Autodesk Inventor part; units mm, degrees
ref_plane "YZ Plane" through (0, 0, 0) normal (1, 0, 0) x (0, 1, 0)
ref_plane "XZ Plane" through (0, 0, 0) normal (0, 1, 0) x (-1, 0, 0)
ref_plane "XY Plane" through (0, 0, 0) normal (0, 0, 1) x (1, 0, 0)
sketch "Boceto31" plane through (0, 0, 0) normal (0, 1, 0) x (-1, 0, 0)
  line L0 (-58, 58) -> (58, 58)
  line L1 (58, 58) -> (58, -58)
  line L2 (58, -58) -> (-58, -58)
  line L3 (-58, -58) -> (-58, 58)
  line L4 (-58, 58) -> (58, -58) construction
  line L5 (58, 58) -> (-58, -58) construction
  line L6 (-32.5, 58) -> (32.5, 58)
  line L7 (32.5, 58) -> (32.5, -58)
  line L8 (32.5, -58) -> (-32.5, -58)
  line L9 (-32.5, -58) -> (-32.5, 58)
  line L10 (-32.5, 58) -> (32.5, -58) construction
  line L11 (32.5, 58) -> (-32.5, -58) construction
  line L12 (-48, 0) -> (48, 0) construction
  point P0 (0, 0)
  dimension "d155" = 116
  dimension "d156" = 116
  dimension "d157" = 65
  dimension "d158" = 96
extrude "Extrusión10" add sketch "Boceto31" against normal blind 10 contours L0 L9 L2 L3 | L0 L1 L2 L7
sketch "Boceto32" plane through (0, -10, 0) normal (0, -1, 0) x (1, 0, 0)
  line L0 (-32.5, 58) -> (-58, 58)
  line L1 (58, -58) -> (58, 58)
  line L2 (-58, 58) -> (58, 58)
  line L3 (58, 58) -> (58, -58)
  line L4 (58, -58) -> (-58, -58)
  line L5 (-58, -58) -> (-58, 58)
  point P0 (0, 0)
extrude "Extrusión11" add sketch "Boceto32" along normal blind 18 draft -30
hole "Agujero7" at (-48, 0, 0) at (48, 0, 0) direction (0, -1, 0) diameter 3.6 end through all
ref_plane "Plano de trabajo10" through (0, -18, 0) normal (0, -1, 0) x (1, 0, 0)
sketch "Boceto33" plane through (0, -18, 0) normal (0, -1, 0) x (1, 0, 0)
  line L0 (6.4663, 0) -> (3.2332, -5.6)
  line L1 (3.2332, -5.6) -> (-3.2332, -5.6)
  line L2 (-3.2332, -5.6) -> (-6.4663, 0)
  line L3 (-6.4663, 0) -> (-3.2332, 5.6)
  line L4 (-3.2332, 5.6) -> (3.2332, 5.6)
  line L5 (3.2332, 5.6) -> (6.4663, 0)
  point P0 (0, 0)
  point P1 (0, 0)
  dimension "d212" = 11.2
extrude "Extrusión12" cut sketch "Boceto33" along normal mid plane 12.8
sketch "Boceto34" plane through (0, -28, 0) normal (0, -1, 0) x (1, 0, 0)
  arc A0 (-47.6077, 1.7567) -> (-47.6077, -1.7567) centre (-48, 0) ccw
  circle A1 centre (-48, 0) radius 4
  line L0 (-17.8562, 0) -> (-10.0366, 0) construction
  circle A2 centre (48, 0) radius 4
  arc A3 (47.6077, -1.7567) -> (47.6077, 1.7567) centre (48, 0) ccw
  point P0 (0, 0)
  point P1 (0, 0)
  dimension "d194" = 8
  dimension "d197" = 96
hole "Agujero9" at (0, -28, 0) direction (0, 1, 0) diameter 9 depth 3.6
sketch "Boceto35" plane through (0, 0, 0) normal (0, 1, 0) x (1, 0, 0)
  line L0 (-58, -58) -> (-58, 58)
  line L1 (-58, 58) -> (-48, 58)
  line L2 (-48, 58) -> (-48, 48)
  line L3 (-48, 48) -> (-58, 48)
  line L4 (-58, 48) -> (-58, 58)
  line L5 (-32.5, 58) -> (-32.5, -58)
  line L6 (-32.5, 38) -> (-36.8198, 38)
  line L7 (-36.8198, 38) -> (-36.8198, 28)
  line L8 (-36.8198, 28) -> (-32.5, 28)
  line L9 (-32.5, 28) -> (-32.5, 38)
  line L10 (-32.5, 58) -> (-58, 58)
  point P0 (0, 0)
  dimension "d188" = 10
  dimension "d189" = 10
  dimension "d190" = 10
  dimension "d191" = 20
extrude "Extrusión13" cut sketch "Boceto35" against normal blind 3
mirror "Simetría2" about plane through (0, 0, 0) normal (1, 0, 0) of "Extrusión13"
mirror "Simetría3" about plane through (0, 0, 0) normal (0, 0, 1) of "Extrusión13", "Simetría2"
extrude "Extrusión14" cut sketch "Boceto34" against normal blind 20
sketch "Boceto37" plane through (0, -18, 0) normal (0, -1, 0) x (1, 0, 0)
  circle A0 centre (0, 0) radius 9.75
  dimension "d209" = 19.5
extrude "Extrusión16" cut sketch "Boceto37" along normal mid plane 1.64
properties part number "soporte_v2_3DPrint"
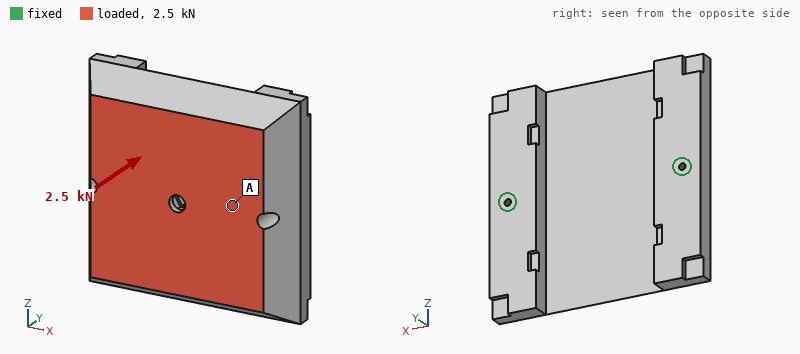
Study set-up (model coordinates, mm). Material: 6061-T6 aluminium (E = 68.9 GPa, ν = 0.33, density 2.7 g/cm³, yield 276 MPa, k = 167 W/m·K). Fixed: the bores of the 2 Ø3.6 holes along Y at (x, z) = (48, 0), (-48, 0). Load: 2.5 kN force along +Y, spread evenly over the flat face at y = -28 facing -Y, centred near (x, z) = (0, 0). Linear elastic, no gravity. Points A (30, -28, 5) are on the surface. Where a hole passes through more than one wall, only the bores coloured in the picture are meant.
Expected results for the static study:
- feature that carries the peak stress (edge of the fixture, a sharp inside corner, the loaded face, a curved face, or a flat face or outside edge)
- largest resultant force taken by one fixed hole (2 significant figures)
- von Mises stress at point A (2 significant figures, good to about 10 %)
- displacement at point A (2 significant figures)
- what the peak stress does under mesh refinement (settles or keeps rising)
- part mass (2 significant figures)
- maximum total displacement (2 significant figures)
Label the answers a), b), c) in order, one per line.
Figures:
a) edge of the fixture
b) 1.6 kN
c) 3.1 MPa
d) 4.3 µm
e) keeps rising
f) 690 g
g) 9.5 µm
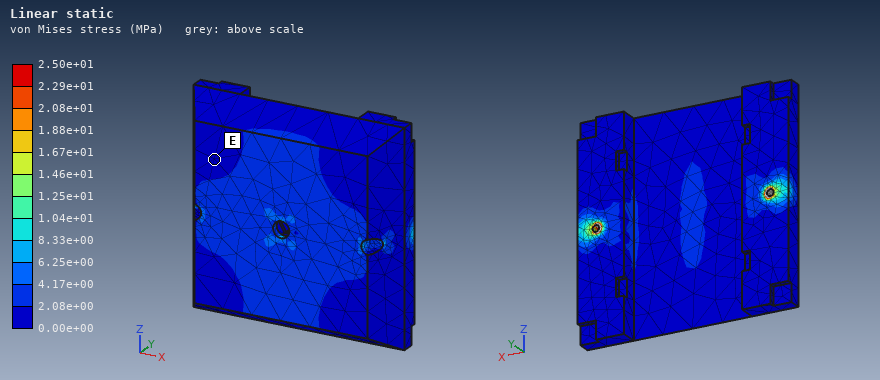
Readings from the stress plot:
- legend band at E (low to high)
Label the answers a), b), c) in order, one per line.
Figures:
a) 0.00e+00 to 2.08e+00 MPa
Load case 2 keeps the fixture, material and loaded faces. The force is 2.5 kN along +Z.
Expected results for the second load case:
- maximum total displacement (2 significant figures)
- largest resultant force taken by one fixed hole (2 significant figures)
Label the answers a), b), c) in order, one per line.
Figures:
a) 0.13 mm
b) 1.3 kN
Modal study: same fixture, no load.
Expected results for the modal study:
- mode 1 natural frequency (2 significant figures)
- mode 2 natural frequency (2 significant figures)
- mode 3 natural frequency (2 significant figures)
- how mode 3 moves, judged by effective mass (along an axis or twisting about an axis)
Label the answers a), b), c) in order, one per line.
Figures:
a) 920 Hz
b) 3700 Hz
c) 4100 Hz
d) along Y
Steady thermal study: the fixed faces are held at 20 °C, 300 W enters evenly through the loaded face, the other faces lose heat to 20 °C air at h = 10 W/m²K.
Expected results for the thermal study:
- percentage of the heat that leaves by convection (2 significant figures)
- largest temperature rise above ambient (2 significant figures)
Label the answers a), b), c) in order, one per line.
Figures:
a) 4.0 %
b) 49 K
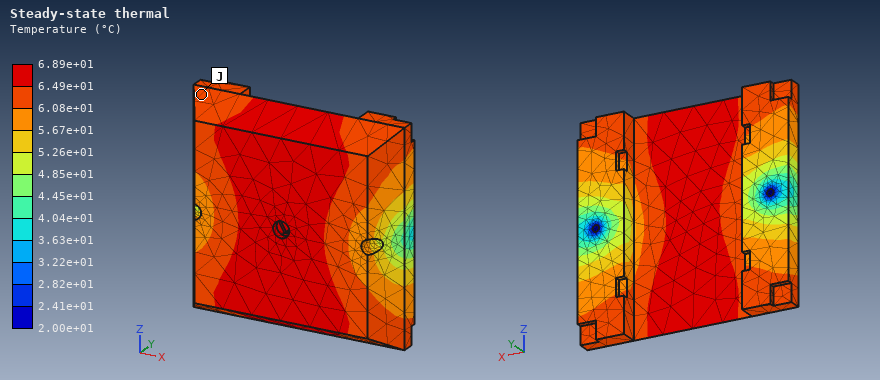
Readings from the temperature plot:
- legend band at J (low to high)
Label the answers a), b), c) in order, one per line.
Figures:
a) 6.08e+01 to 6.49e+01 °C
